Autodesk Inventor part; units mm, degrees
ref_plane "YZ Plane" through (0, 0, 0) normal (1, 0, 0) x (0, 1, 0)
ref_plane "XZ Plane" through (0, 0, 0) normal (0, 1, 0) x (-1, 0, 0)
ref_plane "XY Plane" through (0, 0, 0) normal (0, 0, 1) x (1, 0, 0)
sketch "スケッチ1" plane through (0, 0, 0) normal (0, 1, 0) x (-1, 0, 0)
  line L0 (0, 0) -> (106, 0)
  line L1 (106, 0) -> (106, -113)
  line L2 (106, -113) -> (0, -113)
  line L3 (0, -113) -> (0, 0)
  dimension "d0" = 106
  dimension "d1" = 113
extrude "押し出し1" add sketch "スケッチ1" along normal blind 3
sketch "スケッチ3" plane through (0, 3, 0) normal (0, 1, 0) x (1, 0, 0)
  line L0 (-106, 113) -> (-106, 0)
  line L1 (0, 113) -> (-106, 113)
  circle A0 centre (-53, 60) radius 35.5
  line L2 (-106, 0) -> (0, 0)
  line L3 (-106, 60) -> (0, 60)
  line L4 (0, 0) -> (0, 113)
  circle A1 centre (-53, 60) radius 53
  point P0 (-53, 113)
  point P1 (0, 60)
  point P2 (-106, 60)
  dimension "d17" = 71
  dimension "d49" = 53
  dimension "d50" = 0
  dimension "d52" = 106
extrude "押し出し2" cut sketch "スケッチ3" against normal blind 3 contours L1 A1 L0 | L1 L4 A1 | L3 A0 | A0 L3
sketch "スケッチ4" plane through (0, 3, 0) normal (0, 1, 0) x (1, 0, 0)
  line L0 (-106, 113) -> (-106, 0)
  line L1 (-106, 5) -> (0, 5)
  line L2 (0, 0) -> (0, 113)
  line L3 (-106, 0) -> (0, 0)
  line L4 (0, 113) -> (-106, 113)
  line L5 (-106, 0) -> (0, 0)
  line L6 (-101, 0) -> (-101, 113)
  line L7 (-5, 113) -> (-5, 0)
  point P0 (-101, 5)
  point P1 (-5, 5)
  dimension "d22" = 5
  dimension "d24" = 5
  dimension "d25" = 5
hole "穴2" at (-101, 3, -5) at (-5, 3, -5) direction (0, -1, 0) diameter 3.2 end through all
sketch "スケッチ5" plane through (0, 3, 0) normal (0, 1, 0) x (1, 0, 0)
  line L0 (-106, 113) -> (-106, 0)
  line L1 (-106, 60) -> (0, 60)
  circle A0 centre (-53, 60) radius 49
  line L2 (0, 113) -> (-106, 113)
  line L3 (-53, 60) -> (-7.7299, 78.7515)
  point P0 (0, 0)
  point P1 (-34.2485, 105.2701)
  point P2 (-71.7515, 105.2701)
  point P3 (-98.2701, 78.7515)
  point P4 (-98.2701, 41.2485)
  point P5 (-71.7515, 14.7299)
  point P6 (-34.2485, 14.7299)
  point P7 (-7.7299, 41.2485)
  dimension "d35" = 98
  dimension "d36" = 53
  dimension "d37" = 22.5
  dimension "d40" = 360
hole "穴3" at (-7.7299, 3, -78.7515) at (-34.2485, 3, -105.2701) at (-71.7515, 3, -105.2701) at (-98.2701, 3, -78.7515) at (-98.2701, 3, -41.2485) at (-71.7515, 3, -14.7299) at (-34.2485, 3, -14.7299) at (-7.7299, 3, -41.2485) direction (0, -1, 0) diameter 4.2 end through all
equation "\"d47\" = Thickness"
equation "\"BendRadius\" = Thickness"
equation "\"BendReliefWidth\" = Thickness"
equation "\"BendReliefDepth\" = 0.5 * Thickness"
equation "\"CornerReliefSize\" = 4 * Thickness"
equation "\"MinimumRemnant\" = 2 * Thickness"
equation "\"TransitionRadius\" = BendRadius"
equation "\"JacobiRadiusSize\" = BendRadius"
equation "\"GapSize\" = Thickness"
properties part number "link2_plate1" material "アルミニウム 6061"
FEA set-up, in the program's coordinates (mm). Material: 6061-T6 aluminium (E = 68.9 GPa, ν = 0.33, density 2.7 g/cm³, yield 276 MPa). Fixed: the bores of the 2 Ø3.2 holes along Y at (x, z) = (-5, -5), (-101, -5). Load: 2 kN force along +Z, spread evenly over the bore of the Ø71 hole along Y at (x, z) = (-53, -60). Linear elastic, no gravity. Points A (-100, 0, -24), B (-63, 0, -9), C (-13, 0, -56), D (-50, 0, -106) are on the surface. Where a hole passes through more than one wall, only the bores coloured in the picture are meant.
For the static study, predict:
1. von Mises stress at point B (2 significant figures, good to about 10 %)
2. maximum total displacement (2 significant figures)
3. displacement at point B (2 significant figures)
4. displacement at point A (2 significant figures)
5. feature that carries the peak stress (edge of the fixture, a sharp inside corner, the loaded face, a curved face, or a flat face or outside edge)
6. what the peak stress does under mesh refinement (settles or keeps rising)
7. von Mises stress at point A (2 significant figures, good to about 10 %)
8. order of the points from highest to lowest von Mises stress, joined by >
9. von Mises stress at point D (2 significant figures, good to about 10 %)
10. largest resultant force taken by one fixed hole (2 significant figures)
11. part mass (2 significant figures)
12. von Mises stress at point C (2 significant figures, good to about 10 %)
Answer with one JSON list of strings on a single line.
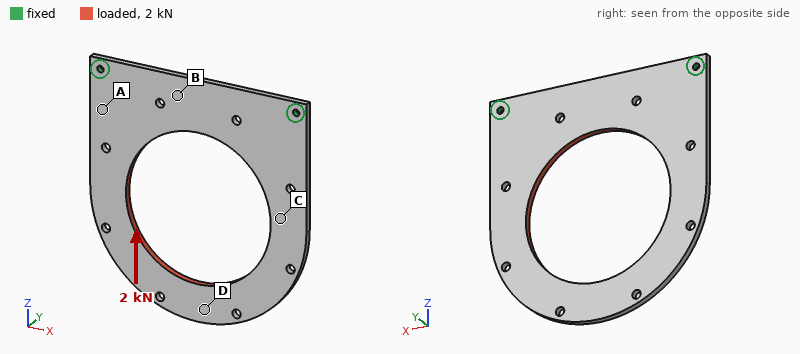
["3.3 MPa", "30 µm", "16 µm", "7.2 µm", "edge of the fixture", "keeps rising", "18 MPa", "A > C > D > B", "7.1 MPa", "1.0 kN", "54 g", "14 MPa"]
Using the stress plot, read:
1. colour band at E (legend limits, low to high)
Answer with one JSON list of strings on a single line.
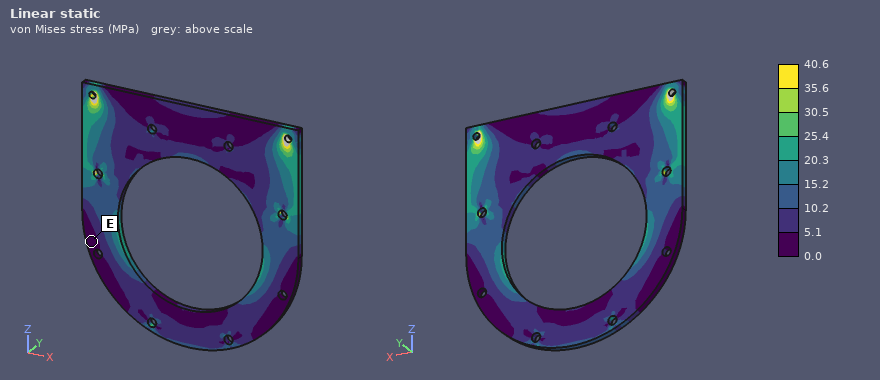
["0.0 to 5.1 MPa"]
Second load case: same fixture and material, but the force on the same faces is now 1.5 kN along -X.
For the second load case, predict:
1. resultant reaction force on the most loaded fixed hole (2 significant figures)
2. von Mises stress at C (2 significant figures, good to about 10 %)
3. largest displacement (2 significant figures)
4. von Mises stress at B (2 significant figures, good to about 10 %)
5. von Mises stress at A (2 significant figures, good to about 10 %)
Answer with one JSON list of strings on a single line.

["1.1 kN", "17 MPa", "0.13 mm", "18 MPa", "22 MPa"]
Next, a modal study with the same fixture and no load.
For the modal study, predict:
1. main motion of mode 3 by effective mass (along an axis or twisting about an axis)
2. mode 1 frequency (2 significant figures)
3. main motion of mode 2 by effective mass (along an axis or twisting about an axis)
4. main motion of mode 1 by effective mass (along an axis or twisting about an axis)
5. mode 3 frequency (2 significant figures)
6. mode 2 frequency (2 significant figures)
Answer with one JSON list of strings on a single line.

["along Y", "200 Hz", "twisting about Z", "along Y", "1100 Hz", "570 Hz"]
